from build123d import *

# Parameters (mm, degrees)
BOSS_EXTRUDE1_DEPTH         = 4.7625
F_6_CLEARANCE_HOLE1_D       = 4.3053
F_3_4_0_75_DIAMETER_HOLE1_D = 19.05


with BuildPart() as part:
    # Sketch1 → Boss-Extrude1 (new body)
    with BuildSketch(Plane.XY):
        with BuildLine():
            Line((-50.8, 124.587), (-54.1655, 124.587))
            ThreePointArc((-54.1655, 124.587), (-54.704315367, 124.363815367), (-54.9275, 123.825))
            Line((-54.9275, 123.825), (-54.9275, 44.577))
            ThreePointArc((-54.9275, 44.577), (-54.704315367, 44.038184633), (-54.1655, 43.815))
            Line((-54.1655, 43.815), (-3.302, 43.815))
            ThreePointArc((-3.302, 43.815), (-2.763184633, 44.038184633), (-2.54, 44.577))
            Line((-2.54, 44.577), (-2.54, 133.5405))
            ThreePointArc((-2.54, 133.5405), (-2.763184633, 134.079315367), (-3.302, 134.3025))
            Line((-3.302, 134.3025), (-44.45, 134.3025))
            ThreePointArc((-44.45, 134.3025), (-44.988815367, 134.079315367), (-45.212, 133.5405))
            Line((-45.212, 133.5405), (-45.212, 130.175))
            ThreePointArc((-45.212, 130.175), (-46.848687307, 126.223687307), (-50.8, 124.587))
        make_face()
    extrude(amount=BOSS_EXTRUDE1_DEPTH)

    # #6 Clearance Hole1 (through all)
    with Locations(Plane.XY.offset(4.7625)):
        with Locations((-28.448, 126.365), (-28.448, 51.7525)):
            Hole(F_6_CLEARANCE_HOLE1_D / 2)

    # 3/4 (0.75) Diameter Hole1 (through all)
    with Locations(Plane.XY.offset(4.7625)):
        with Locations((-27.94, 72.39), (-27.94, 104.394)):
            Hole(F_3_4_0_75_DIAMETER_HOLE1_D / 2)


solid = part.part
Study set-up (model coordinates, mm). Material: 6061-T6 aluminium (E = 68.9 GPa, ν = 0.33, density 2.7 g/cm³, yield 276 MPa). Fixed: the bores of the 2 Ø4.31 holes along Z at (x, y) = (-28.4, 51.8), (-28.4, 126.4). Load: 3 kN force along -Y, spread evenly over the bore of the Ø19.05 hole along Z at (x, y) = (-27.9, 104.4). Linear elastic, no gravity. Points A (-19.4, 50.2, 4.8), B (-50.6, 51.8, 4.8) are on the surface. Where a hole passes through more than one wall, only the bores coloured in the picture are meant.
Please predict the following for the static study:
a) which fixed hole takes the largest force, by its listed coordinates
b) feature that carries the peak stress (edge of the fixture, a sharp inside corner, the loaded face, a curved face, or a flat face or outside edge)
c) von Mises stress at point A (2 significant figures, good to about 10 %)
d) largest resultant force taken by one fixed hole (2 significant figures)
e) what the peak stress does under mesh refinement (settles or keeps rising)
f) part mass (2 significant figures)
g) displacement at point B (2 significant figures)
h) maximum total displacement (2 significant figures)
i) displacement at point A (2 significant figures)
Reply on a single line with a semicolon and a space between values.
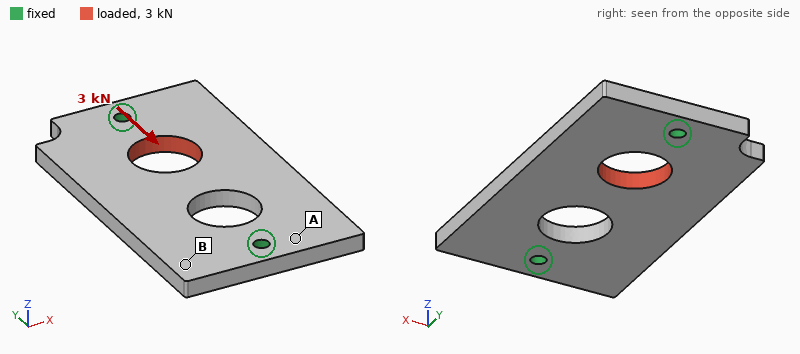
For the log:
(-28.4, 126.4); edge of the fixture; 7.6 MPa; 2.0 kN; keeps rising; 52 g; 6.2 µm; 13 µm; 2.8 µm
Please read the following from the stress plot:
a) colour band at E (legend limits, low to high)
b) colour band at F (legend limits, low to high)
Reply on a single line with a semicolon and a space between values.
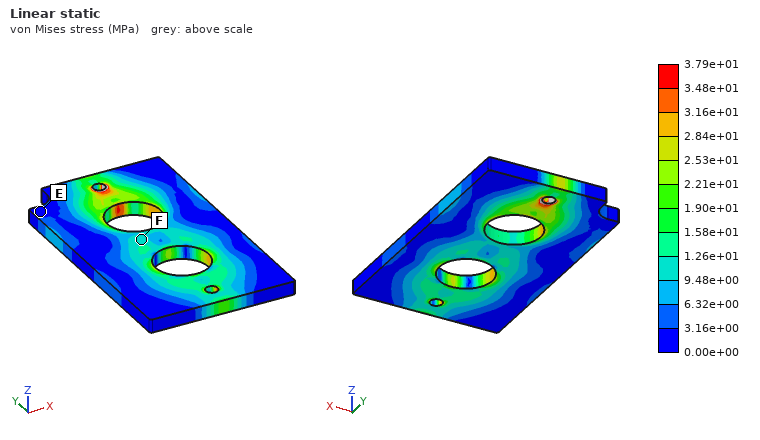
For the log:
0.00e+00 to 3.16e+00 MPa; 9.48e+00 to 1.26e+01 MPa
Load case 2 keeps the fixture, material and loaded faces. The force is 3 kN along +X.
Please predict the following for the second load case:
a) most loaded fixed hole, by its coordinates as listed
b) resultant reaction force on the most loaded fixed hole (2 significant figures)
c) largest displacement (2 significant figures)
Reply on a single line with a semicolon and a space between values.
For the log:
(-28.4, 126.4); 2.1 kN; 18 µm
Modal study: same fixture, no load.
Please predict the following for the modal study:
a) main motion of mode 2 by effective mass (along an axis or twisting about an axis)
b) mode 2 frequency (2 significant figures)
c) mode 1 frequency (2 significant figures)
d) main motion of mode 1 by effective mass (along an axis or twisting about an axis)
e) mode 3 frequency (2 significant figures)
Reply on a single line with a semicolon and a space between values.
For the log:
along Z; 3100 Hz; 2800 Hz; twisting about Y; 5700 Hz
